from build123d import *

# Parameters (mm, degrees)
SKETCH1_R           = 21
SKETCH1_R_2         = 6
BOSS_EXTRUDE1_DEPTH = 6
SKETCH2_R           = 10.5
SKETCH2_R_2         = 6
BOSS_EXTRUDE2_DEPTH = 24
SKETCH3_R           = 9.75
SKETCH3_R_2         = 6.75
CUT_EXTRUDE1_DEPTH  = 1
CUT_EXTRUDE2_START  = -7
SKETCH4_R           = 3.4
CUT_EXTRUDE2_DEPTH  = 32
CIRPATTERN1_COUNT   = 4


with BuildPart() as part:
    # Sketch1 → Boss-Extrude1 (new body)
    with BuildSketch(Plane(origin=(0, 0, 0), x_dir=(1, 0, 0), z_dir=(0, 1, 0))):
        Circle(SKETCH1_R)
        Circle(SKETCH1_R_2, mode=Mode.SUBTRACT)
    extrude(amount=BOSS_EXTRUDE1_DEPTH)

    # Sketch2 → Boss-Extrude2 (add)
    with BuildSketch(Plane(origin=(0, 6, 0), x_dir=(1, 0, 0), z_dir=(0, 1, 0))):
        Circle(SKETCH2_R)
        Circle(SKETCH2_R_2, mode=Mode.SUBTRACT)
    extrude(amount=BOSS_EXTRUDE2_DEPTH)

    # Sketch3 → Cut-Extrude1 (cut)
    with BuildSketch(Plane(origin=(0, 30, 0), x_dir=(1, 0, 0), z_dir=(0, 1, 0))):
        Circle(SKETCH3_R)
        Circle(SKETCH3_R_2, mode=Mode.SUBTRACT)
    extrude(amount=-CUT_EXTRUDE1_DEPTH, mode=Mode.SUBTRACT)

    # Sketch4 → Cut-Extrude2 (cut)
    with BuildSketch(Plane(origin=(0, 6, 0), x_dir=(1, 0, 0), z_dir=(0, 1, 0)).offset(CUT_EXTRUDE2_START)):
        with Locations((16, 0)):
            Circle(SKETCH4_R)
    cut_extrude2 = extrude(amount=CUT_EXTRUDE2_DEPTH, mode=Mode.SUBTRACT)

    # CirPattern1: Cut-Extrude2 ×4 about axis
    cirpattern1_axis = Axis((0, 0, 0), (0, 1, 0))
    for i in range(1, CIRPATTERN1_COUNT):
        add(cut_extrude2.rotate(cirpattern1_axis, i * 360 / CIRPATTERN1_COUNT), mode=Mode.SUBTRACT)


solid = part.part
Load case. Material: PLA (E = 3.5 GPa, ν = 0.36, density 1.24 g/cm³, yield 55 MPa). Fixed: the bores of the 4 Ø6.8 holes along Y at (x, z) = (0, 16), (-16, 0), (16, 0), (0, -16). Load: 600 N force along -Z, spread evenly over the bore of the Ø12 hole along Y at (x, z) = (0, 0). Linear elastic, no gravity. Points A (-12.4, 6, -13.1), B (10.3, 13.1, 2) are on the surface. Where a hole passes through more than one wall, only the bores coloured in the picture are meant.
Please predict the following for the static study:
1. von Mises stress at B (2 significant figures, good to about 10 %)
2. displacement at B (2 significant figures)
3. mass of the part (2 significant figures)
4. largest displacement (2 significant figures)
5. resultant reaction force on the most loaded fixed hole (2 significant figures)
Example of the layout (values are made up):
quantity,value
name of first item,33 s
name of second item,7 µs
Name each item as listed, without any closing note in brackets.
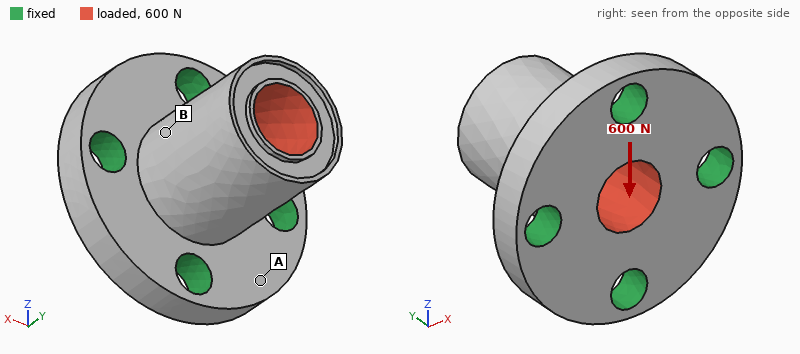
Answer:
quantity,value
von Mises stress at B,3.3 MPa
displacement at B,0.034 mm
mass of the part,15 g
largest displacement,0.11 mm
resultant reaction force on the most loaded fixed hole,330 N
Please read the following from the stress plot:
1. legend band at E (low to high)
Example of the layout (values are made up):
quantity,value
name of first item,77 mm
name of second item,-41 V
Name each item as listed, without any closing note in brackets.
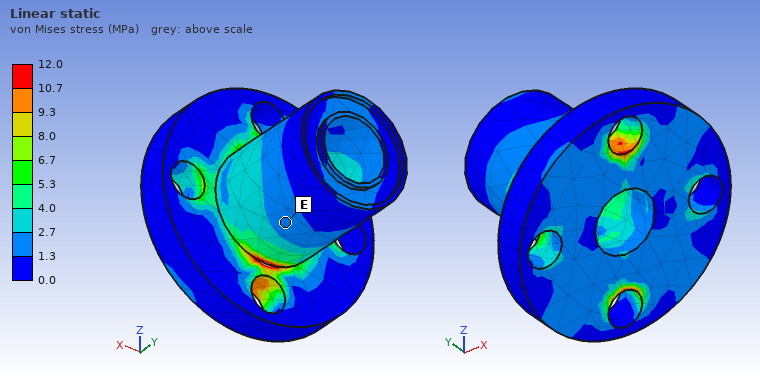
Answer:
quantity,value
legend band at E,1.3 to 2.7 MPa
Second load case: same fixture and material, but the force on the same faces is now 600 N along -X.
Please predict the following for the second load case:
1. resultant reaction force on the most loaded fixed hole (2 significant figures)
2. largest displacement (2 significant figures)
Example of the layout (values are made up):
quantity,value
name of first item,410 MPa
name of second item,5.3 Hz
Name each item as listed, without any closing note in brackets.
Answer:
quantity,value
resultant reaction force on the most loaded fixed hole,330 N
largest displacement,0.11 mm
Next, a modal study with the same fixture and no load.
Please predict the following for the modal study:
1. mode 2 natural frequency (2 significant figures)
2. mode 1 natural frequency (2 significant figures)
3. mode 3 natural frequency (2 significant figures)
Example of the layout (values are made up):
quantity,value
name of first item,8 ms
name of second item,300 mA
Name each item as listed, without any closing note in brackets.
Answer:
quantity,value
mode 2 natural frequency,5000 Hz
mode 1 natural frequency,5000 Hz
mode 3 natural frequency,9800 Hz
